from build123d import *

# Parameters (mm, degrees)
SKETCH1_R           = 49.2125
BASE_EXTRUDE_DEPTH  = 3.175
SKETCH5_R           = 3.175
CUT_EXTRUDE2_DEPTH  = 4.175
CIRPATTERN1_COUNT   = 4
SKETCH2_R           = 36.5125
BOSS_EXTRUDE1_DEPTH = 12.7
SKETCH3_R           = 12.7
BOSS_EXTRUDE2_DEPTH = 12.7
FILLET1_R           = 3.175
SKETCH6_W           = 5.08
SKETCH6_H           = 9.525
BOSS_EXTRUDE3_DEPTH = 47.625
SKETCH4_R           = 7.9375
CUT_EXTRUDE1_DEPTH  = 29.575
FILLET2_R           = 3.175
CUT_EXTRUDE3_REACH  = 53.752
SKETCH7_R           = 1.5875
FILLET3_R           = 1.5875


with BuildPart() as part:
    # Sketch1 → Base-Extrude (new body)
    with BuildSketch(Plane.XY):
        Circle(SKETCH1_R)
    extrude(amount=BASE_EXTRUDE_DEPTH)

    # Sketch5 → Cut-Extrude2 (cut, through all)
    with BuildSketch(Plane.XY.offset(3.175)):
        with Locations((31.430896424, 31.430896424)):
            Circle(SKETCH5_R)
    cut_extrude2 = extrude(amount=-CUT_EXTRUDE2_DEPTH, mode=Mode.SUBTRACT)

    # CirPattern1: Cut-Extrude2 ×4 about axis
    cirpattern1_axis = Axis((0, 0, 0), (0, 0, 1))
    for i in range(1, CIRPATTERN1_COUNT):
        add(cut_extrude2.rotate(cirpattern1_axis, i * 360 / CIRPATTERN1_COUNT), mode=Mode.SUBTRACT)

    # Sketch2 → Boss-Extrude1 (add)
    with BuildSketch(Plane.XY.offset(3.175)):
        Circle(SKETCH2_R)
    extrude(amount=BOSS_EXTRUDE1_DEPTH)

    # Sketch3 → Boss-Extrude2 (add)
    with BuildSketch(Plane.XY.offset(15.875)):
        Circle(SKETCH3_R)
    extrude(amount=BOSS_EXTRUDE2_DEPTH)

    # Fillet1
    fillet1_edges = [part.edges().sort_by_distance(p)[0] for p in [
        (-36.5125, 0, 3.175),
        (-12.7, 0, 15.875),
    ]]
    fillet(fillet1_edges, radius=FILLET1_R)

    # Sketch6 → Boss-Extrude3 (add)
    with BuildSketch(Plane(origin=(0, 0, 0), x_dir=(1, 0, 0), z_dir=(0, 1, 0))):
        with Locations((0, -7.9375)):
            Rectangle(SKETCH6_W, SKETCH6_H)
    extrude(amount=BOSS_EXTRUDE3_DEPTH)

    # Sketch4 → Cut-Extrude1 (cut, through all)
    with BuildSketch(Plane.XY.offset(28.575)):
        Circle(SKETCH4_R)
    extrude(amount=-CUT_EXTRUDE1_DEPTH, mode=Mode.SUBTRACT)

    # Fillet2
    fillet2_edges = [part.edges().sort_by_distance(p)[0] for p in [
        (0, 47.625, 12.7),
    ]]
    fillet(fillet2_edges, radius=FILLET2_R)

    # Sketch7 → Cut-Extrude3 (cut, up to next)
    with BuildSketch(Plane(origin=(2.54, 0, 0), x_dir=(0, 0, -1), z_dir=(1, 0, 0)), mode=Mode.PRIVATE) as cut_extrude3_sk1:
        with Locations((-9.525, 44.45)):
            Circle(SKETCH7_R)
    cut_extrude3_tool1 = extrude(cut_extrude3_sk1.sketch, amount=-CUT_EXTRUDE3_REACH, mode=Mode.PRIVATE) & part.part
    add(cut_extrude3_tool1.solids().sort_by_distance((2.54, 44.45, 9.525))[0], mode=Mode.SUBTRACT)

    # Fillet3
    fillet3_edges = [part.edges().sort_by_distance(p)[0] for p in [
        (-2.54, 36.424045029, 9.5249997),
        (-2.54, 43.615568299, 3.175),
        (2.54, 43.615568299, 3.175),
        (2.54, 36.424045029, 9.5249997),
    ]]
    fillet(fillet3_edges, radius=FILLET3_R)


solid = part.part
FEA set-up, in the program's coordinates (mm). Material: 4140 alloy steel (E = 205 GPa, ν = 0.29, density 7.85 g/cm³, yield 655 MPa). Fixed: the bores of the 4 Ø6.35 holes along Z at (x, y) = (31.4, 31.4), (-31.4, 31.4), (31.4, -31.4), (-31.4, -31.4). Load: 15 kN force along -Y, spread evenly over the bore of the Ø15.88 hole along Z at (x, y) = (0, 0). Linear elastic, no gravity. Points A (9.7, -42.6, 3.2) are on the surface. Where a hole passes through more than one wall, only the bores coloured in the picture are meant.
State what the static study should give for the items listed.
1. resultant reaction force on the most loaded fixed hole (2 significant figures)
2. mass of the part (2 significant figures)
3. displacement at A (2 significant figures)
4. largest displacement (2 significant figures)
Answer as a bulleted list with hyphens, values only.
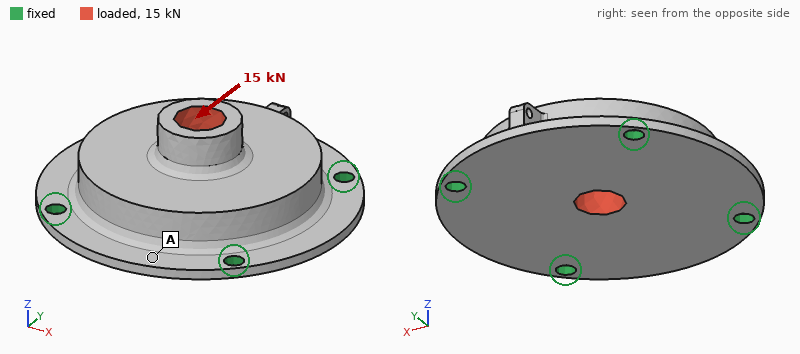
- 4.3 kN
- 620 g
- 11 µm
- 18 µm
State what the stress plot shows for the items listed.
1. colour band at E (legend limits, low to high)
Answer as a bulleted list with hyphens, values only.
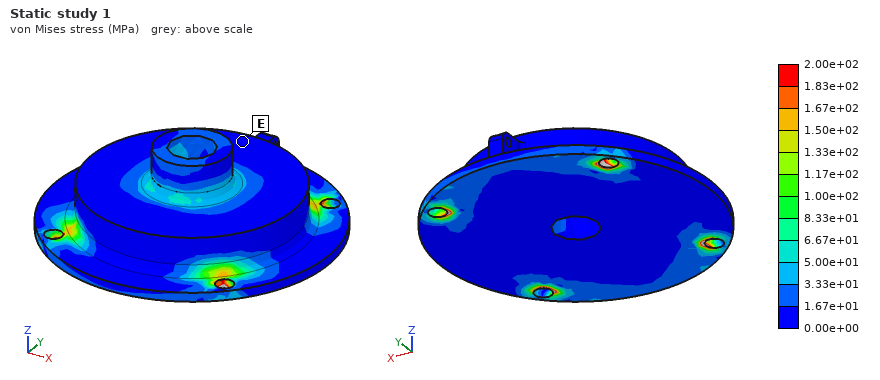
- 0.00e+00 to 1.67e+01 MPa
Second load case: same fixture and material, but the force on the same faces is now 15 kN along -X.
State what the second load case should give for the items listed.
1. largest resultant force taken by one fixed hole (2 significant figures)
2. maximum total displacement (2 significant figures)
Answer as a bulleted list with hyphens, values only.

- 4.3 kN
- 18 µm
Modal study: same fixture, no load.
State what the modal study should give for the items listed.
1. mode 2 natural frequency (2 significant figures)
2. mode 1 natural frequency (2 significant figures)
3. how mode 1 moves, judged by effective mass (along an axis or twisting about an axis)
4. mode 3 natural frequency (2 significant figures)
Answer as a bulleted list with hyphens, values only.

- 7200 Hz
- 5500 Hz
- along Z
- 7300 Hz
